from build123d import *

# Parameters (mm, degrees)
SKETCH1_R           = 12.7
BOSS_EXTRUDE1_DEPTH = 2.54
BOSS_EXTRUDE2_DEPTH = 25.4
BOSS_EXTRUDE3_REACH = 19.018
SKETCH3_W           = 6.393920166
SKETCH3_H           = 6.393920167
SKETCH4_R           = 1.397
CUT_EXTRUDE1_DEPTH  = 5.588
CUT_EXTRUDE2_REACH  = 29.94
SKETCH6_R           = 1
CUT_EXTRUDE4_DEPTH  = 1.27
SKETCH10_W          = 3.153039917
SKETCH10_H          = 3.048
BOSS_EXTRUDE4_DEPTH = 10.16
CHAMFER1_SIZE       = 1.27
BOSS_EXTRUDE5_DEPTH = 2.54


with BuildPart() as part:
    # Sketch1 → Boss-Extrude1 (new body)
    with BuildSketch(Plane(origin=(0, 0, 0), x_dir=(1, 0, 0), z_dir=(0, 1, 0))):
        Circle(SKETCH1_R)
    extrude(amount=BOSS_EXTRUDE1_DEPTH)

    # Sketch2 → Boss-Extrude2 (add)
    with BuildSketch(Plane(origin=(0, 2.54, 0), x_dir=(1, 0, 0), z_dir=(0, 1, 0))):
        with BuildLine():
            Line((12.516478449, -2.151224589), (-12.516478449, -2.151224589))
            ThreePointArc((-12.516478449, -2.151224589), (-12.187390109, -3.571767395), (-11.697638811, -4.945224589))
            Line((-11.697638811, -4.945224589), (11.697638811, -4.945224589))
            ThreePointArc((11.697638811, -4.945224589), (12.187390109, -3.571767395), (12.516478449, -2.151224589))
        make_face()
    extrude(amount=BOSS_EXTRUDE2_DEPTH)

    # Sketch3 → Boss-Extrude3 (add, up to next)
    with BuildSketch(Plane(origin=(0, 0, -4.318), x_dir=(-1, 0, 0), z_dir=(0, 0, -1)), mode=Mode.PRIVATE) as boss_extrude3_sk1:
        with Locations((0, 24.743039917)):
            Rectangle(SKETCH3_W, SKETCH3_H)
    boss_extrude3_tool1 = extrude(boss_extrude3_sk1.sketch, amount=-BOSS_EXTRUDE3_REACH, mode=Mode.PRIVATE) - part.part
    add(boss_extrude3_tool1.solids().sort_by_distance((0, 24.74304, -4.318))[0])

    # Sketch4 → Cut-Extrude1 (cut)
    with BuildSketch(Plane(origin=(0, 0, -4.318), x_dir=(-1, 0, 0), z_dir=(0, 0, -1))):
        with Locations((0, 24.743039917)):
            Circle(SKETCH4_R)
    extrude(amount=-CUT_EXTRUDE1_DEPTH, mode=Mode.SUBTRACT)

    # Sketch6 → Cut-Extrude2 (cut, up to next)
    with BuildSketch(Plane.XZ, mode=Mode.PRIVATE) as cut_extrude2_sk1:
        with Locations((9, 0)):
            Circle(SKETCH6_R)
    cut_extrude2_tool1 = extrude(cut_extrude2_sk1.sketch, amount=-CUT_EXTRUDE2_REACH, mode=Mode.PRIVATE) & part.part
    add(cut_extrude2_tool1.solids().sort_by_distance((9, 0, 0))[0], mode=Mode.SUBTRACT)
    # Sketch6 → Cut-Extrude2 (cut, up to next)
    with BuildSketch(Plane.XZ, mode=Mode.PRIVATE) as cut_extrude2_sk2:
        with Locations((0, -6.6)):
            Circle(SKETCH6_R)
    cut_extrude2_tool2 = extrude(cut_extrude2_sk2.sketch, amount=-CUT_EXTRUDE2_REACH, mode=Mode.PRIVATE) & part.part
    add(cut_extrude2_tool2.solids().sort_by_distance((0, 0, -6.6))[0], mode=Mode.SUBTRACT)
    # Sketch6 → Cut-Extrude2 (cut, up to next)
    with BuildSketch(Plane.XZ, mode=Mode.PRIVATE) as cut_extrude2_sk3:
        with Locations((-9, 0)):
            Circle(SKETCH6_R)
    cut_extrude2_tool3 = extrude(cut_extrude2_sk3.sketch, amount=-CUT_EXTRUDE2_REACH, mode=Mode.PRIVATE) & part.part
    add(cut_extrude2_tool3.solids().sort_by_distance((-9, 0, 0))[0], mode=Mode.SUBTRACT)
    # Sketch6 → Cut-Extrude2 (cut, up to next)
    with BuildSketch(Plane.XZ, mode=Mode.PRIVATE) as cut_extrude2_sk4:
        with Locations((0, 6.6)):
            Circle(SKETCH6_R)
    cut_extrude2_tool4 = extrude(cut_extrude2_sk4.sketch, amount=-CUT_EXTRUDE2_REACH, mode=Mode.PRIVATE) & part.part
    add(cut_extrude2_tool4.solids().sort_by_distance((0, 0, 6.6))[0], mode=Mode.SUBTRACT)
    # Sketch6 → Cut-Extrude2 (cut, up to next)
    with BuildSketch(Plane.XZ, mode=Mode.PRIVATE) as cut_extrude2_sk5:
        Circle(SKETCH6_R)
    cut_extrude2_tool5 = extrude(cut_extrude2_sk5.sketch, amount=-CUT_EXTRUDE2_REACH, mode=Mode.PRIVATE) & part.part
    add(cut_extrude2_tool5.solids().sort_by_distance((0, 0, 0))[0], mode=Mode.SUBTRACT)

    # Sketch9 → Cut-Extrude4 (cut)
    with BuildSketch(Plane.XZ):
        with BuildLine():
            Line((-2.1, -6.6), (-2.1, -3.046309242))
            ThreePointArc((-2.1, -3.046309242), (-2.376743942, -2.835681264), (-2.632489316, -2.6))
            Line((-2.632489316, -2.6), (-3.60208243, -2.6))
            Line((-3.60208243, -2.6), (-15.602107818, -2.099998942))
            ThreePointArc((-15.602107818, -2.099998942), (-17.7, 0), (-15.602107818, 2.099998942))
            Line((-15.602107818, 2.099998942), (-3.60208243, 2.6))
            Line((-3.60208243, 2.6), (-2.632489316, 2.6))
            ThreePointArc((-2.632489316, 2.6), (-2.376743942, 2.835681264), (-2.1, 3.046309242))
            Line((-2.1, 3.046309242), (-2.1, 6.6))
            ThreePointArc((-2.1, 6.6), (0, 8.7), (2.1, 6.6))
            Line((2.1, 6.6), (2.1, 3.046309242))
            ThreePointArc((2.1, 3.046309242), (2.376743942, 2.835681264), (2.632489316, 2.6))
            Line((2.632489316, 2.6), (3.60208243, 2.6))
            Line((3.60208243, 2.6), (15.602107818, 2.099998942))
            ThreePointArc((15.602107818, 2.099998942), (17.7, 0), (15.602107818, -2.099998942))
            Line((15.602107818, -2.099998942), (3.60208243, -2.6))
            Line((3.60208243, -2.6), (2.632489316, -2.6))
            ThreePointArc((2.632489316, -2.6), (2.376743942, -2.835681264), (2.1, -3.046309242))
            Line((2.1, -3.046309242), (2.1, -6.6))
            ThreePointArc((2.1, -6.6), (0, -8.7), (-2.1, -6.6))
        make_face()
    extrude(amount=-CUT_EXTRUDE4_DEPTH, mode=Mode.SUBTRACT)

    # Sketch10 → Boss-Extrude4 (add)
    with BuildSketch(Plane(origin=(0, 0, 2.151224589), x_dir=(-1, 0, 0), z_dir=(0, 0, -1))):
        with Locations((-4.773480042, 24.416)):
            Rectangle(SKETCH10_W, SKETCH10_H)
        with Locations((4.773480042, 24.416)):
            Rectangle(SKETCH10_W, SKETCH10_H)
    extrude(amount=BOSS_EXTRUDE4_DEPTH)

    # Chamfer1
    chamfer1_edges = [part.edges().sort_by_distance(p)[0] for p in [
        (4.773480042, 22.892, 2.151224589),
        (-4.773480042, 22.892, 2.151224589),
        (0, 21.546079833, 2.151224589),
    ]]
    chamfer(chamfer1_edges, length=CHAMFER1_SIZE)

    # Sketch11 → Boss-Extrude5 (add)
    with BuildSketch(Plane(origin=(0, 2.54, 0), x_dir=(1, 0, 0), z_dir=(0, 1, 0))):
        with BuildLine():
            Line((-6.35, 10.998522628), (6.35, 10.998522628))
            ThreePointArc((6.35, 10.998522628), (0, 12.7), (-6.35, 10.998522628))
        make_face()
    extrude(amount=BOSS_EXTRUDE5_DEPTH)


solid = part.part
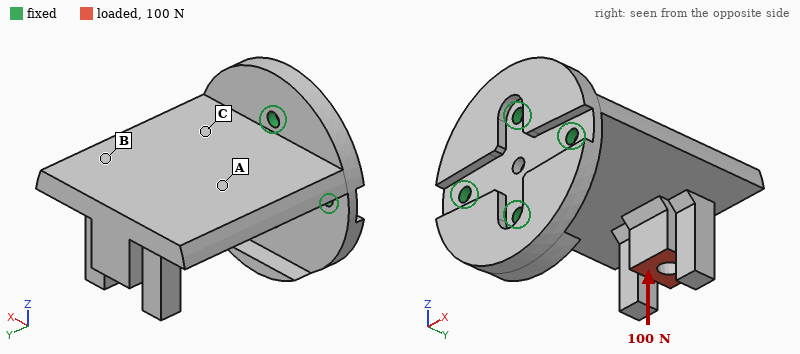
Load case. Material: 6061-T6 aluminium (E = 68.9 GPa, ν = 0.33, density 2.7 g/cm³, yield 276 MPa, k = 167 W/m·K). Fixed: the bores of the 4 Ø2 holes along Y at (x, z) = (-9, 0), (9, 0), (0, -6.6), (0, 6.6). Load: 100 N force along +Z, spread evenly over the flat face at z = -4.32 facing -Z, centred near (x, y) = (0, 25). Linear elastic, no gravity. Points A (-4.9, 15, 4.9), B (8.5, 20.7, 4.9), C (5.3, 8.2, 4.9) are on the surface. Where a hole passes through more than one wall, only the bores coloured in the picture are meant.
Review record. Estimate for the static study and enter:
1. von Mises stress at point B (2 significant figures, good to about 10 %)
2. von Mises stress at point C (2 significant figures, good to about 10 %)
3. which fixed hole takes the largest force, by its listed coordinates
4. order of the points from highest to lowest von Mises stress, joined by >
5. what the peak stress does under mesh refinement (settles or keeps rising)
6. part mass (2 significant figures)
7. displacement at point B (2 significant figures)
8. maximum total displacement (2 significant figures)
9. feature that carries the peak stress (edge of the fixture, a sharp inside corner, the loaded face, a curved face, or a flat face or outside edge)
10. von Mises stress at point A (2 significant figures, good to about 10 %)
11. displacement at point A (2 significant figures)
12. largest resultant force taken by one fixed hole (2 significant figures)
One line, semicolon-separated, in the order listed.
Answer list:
13 MPa; 49 MPa; (0, 6.6); C > A > B; keeps rising; 8.8 g; 0.13 mm; 0.22 mm; edge of the fixture; 30 MPa; 0.077 mm; 380 N
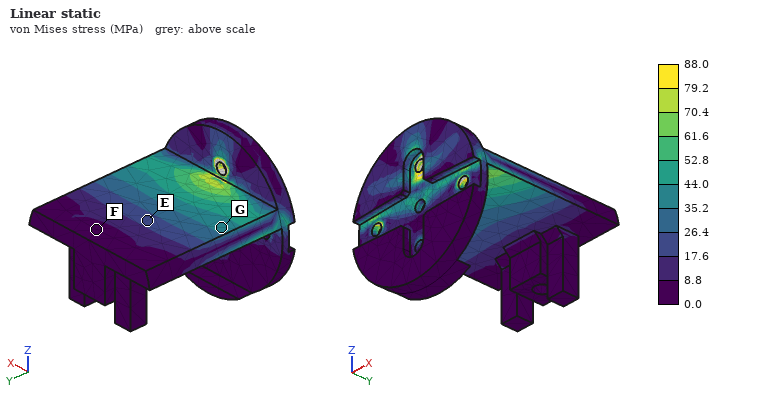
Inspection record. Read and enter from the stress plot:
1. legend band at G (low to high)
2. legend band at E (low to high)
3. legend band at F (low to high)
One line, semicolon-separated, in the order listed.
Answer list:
35.2 to 44.0 MPa; 17.6 to 26.4 MPa; 0.0 to 8.8 MPa
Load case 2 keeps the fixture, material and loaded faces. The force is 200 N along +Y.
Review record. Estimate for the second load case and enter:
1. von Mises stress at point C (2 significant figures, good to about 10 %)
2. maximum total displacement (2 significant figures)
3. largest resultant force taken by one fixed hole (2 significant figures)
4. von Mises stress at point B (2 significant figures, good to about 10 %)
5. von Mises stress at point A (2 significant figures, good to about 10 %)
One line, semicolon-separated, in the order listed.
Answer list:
43 MPa; 0.22 mm; 180 N; 35 MPa; 44 MPa
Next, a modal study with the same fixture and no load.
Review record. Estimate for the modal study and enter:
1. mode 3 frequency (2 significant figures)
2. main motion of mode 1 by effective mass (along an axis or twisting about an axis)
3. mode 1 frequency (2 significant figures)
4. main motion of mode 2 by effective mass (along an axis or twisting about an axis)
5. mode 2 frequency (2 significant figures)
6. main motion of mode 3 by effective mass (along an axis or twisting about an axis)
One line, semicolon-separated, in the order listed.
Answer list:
9200 Hz; along Z; 2200 Hz; along X; 5400 Hz; along X
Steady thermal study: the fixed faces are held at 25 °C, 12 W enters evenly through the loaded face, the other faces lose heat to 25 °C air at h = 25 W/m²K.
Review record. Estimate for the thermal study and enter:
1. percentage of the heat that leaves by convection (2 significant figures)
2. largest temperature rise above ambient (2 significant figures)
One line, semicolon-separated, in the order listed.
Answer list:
8.1 %; 38 K
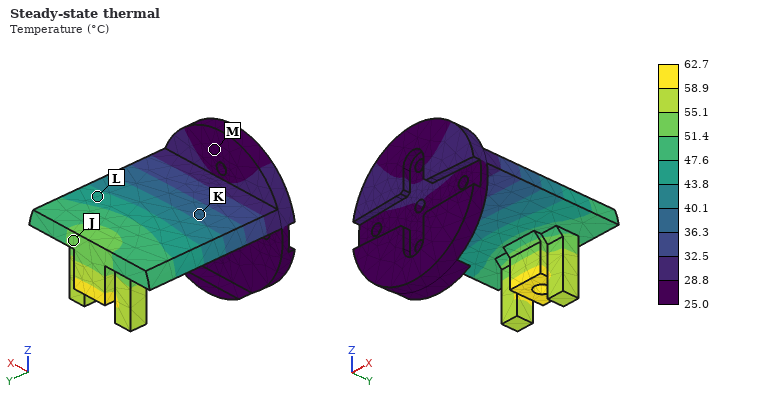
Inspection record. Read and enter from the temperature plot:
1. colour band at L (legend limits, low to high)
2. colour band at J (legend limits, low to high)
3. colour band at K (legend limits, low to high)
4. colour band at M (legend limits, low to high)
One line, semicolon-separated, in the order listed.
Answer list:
43.8 to 47.6 °C; 51.4 to 55.1 °C; 36.3 to 40.1 °C; 25.0 to 28.8 °C
